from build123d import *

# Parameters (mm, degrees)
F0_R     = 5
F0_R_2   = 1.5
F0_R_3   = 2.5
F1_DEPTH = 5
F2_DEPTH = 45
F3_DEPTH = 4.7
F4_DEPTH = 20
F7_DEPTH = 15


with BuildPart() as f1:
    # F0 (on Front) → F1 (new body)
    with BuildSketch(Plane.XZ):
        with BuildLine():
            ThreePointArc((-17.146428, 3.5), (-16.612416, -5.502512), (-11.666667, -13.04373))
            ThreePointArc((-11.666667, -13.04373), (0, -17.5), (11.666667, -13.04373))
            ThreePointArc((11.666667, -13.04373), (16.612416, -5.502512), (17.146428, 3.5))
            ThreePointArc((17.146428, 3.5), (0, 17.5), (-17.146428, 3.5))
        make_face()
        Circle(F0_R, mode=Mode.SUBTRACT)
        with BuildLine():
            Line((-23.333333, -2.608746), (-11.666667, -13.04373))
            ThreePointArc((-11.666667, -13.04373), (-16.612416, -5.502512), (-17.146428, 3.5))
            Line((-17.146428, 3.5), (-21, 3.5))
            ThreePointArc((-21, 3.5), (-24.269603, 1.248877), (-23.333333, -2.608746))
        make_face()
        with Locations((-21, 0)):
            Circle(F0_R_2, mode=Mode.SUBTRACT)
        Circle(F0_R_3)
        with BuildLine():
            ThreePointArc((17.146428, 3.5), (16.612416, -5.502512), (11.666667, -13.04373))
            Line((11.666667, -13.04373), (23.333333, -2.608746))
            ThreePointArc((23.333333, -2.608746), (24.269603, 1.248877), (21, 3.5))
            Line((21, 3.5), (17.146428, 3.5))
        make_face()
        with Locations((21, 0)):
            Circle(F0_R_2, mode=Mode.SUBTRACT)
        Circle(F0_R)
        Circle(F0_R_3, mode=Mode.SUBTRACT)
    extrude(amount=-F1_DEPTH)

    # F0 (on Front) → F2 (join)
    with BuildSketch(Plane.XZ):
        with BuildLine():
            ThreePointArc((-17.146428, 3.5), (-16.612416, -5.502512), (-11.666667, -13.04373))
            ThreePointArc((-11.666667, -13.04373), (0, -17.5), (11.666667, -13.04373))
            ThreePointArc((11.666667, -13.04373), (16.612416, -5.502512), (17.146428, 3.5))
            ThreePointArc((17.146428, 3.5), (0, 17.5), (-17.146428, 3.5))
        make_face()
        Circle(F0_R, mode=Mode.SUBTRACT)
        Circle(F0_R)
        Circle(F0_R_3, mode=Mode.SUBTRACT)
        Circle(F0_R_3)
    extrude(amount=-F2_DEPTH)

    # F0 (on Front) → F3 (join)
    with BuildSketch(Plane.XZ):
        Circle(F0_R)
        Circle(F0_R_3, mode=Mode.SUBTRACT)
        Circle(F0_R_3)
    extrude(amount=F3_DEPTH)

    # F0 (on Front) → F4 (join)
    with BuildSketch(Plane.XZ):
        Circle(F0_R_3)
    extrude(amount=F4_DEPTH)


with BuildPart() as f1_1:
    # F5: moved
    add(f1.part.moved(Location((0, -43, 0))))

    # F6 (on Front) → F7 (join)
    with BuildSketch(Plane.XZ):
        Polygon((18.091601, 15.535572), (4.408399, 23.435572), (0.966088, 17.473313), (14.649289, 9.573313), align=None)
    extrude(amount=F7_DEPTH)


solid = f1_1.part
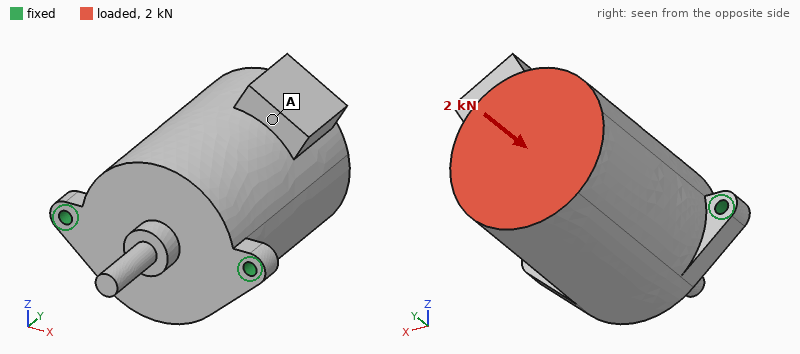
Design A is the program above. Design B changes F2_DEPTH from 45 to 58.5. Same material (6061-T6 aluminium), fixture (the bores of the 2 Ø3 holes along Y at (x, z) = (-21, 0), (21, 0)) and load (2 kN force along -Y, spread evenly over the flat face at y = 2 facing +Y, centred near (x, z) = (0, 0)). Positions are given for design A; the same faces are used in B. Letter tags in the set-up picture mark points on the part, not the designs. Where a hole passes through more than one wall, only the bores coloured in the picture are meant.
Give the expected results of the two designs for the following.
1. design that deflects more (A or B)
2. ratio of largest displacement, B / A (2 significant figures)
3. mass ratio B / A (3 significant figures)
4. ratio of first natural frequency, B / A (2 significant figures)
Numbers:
B
1.1
1.28
0.69
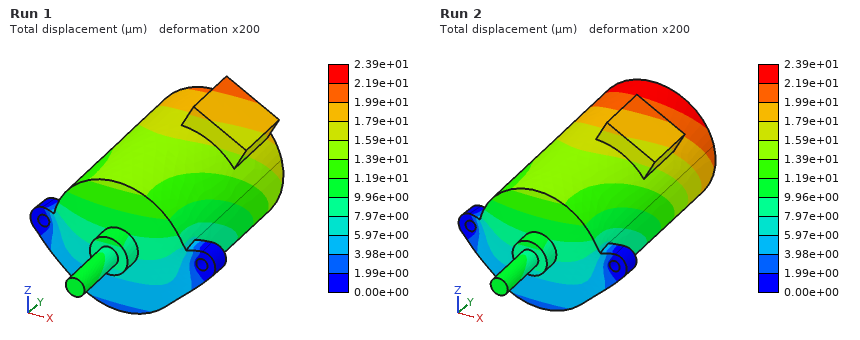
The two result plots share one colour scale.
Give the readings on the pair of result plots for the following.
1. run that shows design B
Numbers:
Run 2
